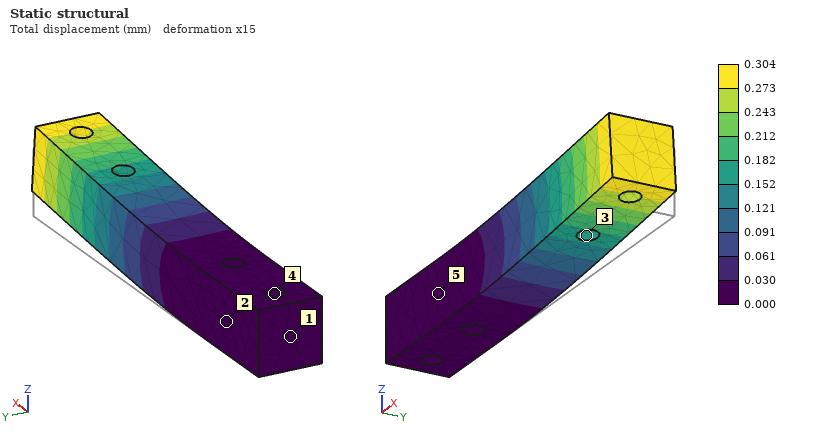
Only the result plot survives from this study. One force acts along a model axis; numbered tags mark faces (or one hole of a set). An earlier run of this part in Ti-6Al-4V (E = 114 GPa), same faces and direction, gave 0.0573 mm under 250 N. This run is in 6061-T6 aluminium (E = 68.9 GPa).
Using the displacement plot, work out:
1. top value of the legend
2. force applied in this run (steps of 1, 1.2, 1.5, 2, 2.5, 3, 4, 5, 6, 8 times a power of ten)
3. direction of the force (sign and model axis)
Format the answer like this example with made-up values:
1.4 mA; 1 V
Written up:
0.304 mm; 800 N; +Z
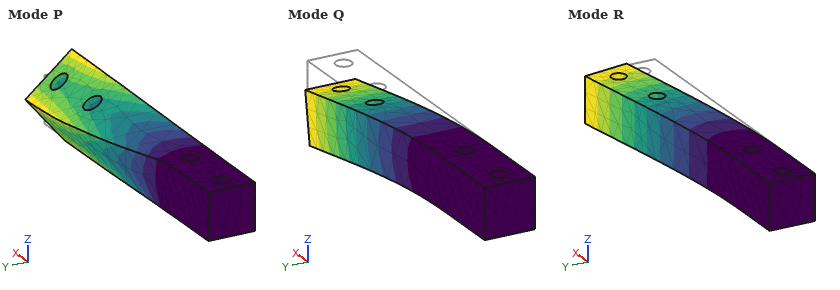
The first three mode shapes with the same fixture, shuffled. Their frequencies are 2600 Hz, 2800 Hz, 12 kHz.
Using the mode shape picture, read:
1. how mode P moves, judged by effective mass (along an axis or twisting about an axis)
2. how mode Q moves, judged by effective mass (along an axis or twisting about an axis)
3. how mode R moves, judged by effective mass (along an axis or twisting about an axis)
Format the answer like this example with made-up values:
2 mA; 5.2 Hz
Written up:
twisting about X; along Z; along Y
